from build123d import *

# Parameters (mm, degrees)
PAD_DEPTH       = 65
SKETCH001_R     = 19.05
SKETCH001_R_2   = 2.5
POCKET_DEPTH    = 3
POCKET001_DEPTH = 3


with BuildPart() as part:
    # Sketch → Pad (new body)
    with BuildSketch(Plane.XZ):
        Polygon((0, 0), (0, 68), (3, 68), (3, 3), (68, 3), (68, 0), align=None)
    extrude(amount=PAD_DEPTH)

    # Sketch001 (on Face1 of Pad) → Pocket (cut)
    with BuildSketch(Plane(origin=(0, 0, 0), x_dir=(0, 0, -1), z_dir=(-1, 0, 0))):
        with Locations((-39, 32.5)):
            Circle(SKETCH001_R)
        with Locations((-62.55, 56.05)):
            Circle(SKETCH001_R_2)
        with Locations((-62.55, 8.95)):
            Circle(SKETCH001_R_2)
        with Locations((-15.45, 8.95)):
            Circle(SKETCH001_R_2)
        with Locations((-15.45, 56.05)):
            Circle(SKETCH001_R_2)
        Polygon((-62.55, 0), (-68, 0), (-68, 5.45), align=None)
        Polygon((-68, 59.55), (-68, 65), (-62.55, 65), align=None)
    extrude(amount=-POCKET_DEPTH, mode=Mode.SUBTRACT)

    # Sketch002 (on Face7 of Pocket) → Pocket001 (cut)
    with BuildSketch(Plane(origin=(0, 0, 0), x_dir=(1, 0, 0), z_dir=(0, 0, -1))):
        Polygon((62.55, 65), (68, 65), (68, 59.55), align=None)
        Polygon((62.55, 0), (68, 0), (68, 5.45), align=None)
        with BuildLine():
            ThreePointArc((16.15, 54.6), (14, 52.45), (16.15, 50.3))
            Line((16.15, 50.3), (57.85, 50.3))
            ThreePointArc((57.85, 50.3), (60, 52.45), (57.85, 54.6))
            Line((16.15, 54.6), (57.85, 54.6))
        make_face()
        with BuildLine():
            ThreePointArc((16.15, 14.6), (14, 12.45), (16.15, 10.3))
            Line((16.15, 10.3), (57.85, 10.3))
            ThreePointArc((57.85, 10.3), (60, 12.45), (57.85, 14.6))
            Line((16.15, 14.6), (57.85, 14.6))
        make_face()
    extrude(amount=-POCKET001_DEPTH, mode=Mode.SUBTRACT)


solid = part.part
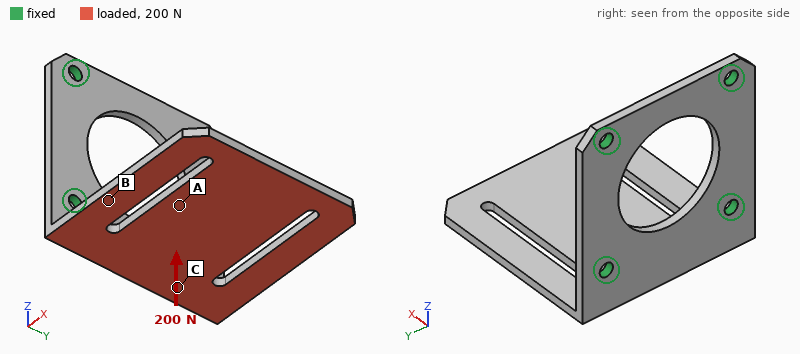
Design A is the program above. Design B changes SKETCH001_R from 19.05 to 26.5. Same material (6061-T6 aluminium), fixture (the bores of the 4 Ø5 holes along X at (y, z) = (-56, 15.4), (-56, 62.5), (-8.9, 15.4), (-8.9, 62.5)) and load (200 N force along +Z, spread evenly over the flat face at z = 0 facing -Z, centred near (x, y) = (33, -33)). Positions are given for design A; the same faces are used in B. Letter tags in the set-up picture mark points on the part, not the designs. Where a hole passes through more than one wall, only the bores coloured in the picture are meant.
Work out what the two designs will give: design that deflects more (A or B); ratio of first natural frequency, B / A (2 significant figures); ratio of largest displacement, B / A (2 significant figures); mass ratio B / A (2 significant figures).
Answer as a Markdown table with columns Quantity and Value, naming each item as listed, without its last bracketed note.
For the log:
| Quantity | Value |
|---|---|
| design that deflects more | B |
| ratio of first natural frequency, B / A | 0.96 |
| ratio of largest displacement, B / A | 1.1 |
| mass ratio B / A | 0.85 |
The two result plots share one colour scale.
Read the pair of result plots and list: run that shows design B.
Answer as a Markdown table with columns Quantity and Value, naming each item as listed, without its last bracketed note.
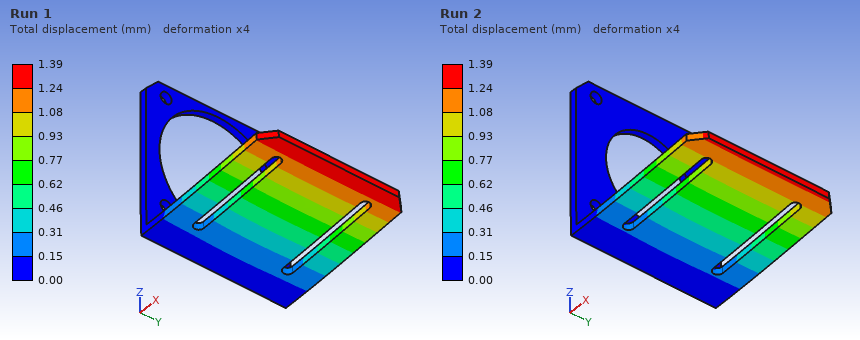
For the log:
| Quantity | Value |
|---|---|
| run that shows design B | Run 1 |
